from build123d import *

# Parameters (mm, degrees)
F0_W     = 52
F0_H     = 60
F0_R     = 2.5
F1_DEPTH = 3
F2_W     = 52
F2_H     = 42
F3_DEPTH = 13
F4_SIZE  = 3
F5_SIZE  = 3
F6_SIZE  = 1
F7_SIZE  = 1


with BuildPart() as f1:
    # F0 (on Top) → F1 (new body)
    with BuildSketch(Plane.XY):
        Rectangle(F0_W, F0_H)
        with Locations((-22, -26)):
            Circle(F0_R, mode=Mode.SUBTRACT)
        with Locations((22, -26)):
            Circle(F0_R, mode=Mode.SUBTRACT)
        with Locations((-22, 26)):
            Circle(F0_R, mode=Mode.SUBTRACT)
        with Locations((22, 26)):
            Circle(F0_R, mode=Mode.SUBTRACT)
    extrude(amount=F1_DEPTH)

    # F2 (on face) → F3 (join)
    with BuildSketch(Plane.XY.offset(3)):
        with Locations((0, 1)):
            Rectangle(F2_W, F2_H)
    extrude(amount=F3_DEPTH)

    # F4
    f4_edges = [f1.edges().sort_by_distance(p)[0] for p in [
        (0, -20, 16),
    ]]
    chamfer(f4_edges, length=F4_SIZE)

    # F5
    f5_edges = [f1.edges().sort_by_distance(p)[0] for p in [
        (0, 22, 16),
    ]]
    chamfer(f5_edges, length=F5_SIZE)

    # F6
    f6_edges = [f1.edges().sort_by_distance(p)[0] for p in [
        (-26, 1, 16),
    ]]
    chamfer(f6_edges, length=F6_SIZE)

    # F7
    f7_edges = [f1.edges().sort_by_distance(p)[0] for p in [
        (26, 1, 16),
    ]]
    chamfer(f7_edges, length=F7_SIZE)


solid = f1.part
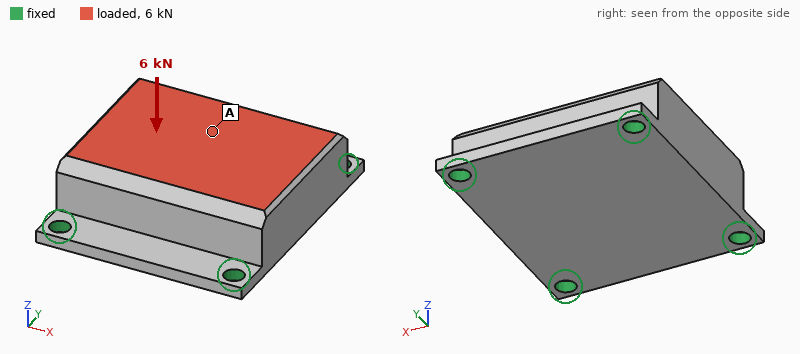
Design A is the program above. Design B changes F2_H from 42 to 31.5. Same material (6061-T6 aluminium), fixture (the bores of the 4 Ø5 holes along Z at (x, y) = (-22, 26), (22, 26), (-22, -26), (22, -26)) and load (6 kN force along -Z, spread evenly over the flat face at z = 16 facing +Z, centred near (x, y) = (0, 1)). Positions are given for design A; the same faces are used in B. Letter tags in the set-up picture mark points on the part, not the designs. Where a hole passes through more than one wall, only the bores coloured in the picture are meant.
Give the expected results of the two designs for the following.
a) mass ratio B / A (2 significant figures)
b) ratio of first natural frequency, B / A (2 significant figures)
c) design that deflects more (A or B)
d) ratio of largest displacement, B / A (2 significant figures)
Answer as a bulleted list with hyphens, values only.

- 0.81
- 0.62
- B
- 3.2
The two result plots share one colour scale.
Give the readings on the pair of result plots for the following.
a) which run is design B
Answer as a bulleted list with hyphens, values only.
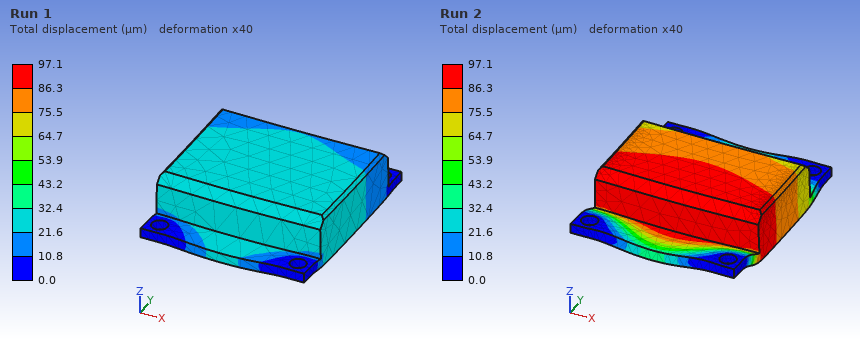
- Run 2
